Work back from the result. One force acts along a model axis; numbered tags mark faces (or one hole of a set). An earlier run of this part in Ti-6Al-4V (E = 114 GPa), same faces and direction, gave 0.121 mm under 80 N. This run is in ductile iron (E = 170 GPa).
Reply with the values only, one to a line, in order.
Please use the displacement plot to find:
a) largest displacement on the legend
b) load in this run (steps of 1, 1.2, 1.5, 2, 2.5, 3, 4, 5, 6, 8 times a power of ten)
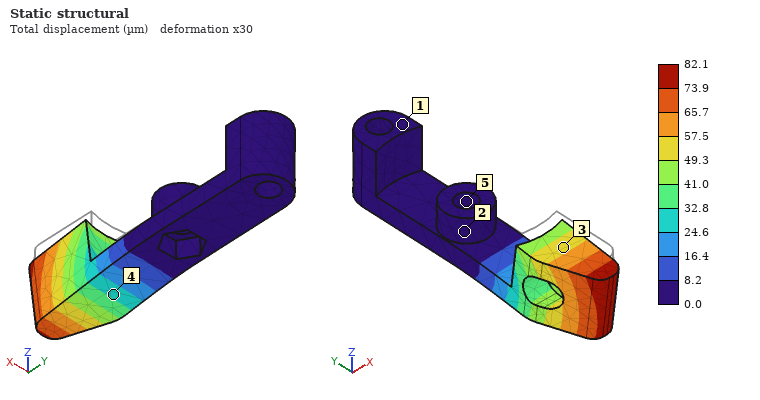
82.1 µm
80 N
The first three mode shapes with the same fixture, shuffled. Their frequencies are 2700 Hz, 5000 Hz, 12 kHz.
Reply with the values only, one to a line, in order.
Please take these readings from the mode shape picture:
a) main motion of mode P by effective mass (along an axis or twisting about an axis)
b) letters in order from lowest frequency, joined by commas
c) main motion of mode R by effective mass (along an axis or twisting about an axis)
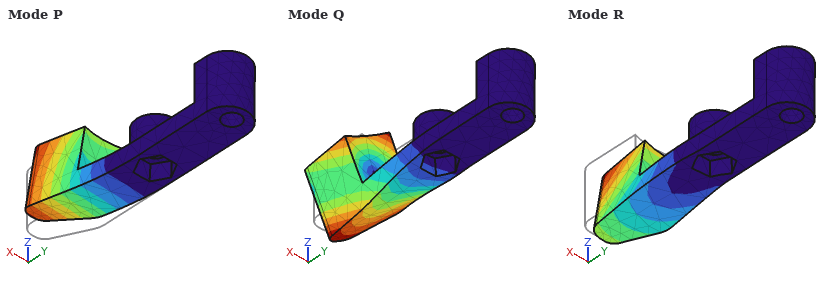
along Z
P, R, Q
along X
